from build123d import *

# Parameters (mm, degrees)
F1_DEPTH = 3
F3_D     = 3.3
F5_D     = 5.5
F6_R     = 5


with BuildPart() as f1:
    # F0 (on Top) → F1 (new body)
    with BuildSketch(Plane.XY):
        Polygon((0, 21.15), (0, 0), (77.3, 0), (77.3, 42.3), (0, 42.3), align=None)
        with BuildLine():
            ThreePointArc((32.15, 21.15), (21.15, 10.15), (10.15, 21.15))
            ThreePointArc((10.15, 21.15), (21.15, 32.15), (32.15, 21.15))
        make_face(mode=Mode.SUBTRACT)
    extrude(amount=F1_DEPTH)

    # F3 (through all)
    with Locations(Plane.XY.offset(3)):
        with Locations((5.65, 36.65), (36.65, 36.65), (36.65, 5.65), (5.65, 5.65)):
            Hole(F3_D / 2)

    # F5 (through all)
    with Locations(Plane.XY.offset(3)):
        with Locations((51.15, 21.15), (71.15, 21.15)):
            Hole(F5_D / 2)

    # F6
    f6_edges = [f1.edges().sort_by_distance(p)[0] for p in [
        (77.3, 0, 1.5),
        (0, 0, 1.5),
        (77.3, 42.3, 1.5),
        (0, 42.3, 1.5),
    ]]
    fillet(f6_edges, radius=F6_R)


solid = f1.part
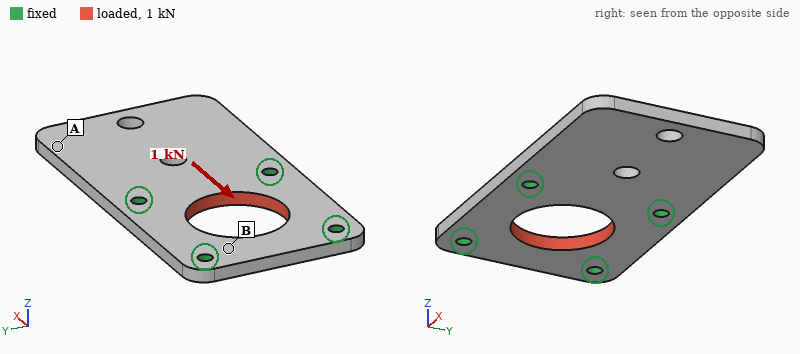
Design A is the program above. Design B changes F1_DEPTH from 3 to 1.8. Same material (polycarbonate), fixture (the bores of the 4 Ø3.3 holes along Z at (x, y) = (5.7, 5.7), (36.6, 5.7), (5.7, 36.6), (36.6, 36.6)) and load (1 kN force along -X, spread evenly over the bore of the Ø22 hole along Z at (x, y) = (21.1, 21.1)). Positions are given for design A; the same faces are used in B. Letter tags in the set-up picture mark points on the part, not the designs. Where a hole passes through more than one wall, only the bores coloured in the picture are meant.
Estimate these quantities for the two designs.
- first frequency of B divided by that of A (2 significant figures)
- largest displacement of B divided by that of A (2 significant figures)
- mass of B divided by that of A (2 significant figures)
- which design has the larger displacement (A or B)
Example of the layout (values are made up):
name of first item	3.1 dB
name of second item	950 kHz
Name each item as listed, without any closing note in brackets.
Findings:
first frequency of B divided by that of A	0.62
largest displacement of B divided by that of A	1.7
mass of B divided by that of A	0.60
which design has the larger displacement	B
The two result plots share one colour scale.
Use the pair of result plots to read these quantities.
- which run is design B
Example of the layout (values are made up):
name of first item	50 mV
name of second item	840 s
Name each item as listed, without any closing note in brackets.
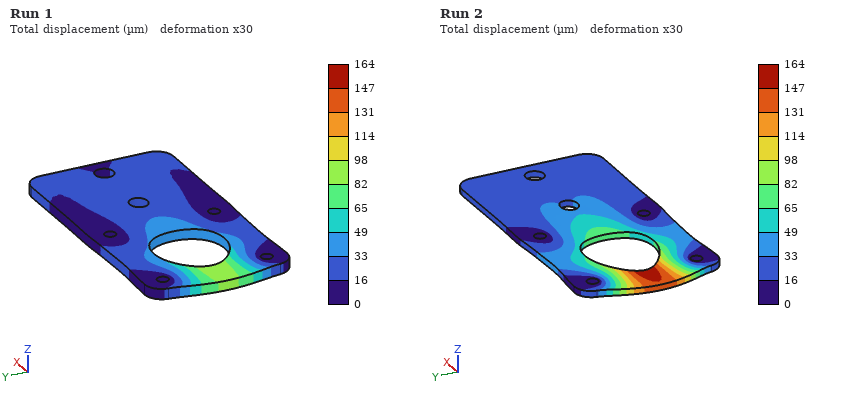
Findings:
which run is design B	Run 2
